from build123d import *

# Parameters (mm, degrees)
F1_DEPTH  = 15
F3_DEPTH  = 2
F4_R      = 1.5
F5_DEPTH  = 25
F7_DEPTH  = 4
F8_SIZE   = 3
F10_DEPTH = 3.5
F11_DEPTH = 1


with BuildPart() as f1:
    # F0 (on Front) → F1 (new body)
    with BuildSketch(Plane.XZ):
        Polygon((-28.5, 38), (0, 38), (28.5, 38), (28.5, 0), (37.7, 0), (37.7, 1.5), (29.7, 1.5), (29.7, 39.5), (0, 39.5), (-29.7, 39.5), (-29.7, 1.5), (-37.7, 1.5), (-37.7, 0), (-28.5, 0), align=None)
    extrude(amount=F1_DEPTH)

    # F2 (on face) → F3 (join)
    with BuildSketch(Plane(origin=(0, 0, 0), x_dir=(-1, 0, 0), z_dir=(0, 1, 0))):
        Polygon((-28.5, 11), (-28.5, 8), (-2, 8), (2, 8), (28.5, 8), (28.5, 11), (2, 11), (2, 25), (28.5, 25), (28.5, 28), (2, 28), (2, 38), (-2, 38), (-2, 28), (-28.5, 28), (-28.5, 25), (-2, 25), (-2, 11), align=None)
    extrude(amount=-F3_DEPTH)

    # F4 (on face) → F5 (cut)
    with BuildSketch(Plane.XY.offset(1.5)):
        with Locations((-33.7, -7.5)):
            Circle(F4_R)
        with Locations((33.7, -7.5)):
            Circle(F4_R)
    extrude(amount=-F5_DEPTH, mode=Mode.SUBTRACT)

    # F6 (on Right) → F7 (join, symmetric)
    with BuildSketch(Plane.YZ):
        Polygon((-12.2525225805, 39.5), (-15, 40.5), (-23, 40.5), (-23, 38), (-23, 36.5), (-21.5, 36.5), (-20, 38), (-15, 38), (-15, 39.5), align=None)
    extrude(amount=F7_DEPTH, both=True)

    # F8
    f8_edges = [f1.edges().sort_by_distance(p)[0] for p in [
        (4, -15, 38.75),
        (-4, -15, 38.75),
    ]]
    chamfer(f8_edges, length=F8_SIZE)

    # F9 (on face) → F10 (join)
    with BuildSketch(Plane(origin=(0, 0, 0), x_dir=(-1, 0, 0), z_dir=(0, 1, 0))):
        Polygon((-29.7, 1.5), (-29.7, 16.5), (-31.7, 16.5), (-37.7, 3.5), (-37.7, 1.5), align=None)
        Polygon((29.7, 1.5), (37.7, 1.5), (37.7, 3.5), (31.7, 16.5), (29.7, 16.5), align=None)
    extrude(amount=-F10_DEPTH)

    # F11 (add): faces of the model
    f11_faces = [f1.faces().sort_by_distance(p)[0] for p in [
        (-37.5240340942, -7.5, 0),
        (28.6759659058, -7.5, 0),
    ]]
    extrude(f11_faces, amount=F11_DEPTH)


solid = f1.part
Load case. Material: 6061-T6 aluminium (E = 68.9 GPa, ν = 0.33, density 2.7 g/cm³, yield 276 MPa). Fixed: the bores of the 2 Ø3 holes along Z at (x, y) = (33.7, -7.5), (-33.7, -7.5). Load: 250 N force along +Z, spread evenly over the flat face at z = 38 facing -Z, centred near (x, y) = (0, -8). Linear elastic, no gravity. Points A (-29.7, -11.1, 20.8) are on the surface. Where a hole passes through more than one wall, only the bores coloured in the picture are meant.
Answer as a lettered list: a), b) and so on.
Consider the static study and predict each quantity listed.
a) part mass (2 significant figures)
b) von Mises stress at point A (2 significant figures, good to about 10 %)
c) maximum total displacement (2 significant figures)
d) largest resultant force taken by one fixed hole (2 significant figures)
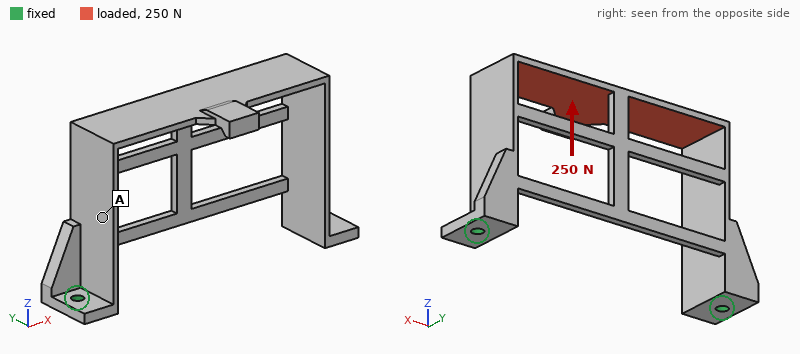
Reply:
a) 13 g
b) 13 MPa
c) 0.50 mm
d) 130 N
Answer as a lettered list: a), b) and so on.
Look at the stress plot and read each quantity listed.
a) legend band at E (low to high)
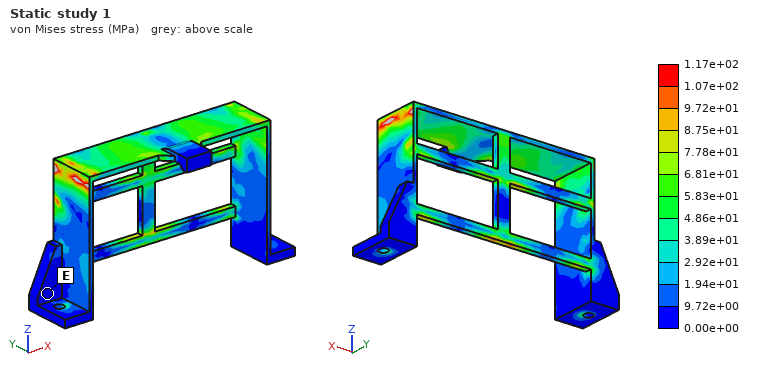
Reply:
a) 0.00e+00 to 9.72e+00 MPa
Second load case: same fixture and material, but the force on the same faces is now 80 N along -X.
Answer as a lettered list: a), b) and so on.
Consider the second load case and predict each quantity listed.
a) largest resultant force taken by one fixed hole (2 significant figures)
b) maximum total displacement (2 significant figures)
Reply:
a) 51 N
b) 0.13 mm
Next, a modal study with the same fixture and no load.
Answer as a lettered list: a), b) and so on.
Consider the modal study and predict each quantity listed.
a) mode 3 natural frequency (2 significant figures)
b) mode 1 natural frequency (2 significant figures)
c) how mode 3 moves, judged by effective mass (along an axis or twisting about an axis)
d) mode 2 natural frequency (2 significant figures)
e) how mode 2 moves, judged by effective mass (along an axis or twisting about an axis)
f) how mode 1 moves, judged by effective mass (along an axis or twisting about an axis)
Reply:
a) 2000 Hz
b) 1600 Hz
c) along Z
d) 1700 Hz
e) along X
f) along Y
